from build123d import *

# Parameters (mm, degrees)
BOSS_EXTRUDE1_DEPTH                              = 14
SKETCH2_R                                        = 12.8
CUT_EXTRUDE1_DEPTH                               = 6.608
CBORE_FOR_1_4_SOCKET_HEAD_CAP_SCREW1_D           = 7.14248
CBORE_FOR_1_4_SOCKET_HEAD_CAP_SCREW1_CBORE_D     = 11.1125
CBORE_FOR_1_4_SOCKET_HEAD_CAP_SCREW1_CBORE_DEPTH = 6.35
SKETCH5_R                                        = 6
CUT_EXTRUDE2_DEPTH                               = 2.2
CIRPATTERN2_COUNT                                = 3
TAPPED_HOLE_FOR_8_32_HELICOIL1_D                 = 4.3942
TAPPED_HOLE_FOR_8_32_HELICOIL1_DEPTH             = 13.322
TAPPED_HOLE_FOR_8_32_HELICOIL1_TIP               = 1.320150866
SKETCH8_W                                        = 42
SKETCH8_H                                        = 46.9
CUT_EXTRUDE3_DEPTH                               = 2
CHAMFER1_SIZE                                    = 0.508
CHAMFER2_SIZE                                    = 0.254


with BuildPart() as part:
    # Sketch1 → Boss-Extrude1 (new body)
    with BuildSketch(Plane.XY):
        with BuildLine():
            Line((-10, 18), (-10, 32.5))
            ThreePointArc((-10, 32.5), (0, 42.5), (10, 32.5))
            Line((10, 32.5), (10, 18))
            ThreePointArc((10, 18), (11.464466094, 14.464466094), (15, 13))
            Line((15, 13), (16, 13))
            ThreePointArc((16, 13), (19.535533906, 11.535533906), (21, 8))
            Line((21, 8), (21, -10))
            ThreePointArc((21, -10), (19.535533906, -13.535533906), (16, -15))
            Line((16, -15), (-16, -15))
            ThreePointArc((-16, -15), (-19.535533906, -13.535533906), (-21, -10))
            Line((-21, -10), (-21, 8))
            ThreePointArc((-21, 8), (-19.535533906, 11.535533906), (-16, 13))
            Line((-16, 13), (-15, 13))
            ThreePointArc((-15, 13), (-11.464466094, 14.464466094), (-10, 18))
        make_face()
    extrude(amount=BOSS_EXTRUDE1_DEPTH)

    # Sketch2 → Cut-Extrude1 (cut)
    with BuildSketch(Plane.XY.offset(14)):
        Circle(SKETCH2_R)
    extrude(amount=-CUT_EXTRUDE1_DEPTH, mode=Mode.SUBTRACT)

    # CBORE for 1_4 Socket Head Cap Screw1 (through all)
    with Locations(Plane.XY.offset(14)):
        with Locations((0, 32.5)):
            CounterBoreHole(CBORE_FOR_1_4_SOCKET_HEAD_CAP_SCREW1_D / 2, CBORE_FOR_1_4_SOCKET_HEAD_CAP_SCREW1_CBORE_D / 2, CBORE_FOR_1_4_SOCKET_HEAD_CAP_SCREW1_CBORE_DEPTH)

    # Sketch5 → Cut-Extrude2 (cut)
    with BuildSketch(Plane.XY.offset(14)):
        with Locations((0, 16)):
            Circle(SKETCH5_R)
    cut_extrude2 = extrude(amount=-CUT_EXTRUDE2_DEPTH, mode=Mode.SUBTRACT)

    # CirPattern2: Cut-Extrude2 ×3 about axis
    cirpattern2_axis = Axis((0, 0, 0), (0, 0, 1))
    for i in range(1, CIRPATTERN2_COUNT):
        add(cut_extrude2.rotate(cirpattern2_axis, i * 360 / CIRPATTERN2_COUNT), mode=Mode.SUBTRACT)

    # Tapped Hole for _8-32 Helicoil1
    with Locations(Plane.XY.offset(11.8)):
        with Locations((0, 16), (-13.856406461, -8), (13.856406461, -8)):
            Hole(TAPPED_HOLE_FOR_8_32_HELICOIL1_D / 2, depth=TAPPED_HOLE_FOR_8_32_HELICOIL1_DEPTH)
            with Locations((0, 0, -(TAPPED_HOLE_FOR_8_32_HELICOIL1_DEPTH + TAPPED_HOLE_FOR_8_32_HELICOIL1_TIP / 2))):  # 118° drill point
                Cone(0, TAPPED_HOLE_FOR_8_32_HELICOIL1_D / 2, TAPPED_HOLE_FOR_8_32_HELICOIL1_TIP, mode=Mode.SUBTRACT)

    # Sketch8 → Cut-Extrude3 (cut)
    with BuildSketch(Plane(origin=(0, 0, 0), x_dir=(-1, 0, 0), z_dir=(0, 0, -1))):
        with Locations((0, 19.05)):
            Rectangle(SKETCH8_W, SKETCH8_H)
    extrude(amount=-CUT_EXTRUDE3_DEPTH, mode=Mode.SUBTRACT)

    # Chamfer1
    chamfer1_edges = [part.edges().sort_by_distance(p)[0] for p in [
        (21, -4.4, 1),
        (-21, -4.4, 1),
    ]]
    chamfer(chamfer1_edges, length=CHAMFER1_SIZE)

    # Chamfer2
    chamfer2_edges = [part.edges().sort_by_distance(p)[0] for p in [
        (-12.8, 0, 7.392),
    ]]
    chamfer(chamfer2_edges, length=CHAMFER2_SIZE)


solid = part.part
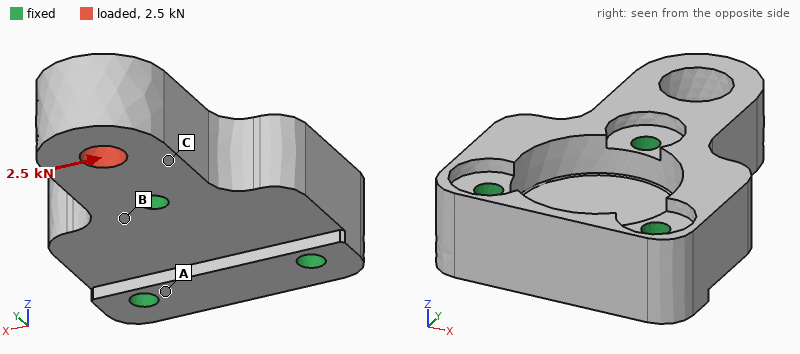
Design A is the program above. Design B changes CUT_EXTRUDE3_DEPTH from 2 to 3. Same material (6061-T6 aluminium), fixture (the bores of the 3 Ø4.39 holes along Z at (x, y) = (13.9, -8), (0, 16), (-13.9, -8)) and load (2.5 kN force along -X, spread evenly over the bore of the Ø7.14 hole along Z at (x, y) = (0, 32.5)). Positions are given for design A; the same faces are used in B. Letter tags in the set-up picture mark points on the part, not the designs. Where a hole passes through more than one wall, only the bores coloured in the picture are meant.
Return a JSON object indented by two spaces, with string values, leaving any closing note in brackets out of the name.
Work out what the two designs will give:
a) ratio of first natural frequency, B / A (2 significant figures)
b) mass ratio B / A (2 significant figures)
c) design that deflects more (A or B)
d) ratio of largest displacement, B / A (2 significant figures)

{
  "ratio of first natural frequency, B / A": "0.93",
  "mass ratio B / A": "0.92",
  "design that deflects more": "B",
  "ratio of largest displacement, B / A": "1.1"
}
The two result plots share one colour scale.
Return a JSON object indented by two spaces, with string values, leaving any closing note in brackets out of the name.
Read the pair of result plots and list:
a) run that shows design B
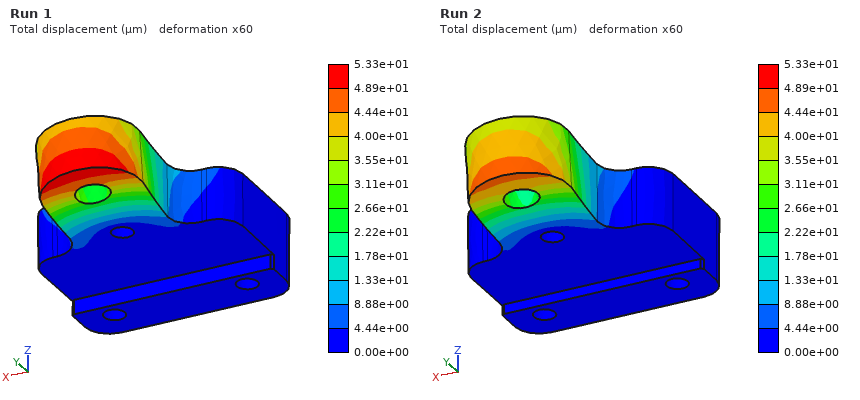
{
  "run that shows design B": "Run 1"
}
